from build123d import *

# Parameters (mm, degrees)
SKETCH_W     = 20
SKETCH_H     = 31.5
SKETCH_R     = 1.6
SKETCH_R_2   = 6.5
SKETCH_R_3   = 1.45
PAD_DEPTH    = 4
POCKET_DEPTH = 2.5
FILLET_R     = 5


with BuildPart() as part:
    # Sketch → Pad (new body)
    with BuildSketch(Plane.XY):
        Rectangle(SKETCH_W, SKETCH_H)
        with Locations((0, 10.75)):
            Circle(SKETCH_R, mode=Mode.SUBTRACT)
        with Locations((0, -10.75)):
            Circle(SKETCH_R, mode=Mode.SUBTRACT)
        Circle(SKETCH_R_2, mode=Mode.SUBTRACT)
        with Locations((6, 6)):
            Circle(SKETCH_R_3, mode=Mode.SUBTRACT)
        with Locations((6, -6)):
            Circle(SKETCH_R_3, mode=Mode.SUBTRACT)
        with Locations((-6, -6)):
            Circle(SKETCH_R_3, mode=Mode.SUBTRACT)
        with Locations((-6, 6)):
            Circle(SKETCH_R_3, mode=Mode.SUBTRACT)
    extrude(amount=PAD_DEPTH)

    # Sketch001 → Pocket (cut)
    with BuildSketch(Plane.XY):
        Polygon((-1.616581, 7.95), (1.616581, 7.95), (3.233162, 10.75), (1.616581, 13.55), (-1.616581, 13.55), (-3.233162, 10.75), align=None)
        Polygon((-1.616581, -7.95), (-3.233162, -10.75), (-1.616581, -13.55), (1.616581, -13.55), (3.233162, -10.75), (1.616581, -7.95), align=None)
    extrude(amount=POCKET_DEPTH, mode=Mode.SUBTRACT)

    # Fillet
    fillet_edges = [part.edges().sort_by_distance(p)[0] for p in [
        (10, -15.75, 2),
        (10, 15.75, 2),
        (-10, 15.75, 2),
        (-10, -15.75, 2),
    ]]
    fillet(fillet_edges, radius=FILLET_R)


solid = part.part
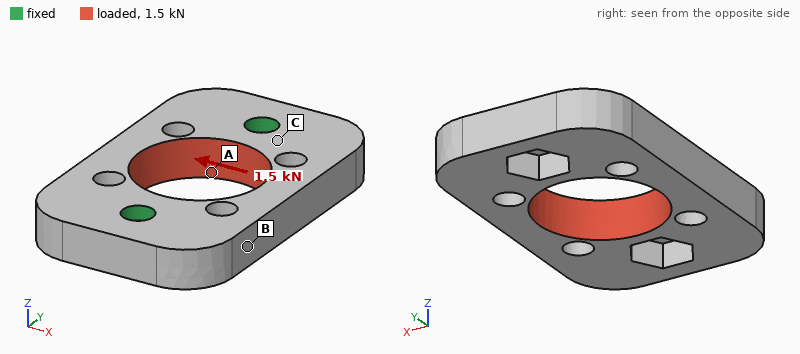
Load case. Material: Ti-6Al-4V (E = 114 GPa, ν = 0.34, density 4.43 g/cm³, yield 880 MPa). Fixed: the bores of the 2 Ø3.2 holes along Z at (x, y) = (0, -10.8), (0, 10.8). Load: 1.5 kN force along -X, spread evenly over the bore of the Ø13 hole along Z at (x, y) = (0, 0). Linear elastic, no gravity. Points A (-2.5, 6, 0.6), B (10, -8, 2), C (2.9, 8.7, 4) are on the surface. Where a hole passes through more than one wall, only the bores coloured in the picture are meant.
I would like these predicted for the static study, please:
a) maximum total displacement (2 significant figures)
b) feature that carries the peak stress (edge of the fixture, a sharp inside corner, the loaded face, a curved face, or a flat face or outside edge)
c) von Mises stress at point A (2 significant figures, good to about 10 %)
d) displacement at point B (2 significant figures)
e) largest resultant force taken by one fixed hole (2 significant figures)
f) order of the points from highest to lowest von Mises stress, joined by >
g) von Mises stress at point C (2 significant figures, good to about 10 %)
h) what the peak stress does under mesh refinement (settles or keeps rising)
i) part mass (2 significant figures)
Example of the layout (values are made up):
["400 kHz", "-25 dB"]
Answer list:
["19 µm", "edge of the fixture", "55 MPa", "15 µm", "750 N", "A > C > B", "42 MPa", "keeps rising", "7.3 g"]
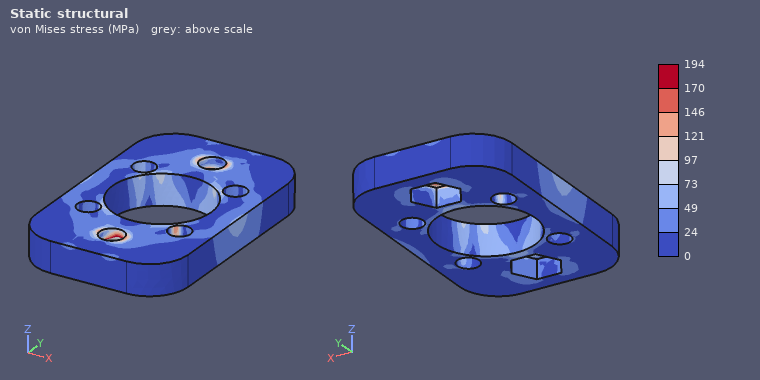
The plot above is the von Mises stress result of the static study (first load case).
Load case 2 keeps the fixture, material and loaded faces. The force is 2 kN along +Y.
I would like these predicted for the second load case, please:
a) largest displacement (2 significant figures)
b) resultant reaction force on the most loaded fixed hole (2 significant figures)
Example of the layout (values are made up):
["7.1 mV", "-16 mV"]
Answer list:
["7.6 µm", "1.0 kN"]
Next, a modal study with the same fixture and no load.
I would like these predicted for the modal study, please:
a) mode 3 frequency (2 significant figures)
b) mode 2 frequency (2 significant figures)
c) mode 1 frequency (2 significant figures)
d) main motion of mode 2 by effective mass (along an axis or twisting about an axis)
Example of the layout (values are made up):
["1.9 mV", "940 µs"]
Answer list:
["19 kHz", "18 kHz", "11 kHz", "along Z"]
